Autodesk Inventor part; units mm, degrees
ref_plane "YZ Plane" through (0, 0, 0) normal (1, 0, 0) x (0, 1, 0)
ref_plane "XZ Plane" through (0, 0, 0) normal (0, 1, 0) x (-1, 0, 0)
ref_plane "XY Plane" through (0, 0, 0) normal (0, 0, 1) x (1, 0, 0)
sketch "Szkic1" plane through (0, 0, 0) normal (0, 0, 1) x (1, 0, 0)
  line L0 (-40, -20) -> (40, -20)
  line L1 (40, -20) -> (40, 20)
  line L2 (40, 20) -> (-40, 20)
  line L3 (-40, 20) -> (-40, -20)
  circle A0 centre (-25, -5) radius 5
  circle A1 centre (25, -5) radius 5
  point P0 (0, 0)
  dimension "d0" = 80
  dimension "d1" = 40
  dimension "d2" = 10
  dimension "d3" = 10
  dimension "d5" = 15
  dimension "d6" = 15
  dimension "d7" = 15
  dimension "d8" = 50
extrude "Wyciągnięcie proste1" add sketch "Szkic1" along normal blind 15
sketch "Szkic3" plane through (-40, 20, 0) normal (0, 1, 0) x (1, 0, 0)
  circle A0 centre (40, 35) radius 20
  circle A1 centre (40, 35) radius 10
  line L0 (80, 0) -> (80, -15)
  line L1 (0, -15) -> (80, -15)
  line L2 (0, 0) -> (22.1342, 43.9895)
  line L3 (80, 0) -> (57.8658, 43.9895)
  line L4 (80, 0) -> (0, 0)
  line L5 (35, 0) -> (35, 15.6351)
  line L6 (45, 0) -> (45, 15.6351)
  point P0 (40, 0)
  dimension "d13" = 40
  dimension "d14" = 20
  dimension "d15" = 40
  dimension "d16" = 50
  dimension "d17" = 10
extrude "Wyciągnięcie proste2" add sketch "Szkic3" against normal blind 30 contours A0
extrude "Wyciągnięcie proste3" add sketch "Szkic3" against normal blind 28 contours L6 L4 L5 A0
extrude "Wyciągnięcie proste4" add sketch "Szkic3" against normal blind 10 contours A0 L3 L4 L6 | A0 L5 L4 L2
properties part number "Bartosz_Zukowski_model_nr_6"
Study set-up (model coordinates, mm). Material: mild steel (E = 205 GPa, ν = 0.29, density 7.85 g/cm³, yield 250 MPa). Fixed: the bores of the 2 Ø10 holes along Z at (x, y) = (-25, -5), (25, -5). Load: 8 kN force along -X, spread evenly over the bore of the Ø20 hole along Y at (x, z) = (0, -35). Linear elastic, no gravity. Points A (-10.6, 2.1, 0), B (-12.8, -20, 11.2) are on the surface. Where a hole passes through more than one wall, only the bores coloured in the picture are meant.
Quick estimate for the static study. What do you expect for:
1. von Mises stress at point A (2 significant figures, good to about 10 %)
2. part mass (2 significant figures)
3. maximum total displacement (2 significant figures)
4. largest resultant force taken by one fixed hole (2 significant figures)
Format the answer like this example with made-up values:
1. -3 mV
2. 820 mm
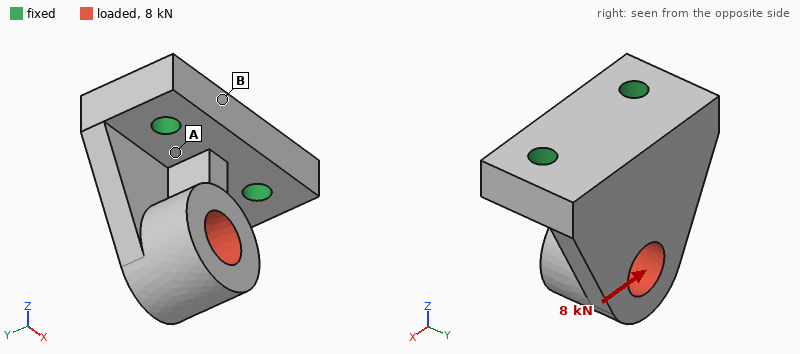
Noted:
1. 38 MPa
2. 730 g
3. 42 µm
4. 7.5 kN
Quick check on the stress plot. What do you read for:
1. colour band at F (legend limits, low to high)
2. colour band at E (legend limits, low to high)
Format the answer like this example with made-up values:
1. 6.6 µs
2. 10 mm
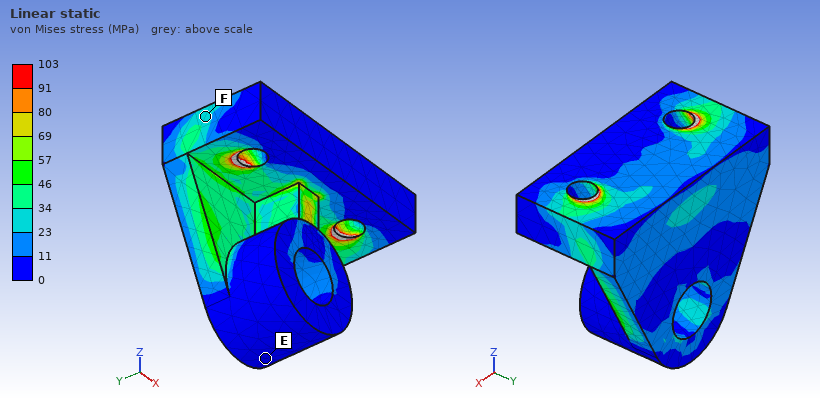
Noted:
1. 23 to 34 MPa
2. 0 to 11 MPa
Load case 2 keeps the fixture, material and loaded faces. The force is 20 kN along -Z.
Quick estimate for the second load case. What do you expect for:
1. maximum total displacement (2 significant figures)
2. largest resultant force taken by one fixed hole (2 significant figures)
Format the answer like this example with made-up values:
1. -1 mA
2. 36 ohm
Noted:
1. 29 µm
2. 10 kN
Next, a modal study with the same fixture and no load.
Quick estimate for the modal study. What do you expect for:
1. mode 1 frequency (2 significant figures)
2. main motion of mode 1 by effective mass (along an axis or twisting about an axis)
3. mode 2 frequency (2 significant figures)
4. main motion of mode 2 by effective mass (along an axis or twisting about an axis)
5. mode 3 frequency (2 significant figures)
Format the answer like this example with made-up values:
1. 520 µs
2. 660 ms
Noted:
1. 3100 Hz
2. along Y
3. 5100 Hz
4. along X
5. 8800 Hz
